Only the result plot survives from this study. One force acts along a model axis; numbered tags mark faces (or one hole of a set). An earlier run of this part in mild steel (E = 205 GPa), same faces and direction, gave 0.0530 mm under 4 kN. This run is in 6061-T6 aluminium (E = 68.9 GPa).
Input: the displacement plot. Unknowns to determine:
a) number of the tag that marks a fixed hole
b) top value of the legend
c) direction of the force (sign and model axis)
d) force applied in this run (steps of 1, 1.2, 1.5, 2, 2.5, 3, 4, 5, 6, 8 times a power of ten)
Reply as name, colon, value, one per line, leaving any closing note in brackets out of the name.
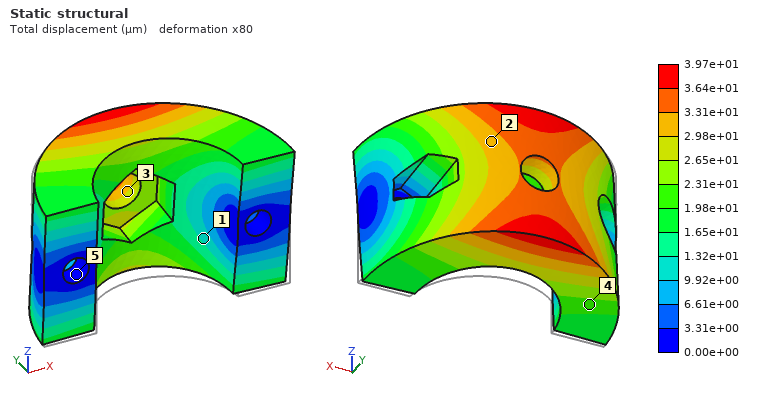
number of the tag that marks a fixed hole: 5
top value of the legend: 3.97e+01 µm
direction of the force: +Z
force applied in this run: 1 kN
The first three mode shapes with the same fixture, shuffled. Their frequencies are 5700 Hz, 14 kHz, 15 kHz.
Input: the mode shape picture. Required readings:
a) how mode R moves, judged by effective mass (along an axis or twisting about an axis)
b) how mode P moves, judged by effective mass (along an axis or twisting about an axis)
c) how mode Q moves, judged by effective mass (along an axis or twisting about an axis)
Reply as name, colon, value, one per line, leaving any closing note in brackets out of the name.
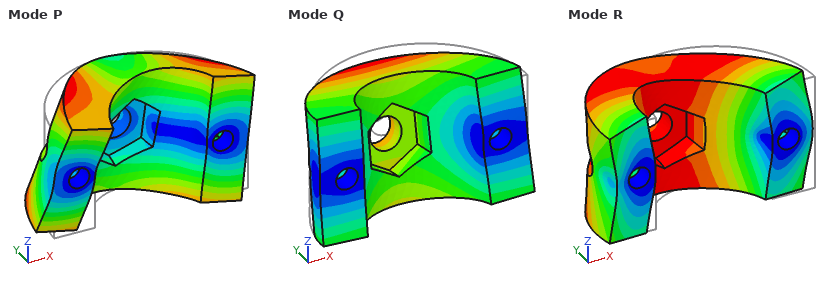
how mode R moves, judged by effective mass: along X
how mode P moves, judged by effective mass: twisting about Y
how mode Q moves, judged by effective mass: along Z
